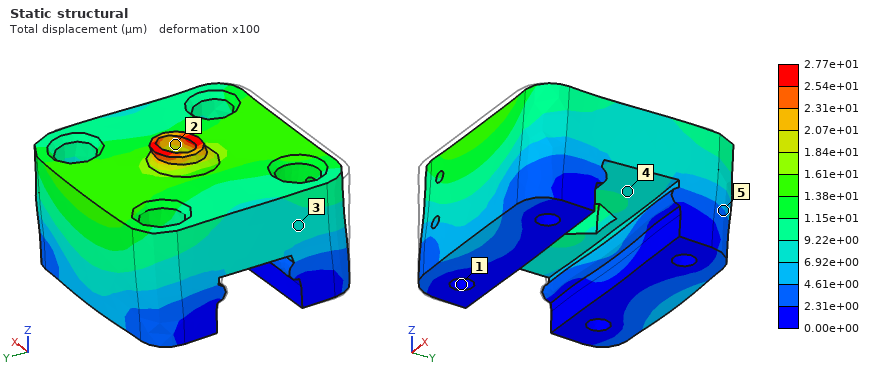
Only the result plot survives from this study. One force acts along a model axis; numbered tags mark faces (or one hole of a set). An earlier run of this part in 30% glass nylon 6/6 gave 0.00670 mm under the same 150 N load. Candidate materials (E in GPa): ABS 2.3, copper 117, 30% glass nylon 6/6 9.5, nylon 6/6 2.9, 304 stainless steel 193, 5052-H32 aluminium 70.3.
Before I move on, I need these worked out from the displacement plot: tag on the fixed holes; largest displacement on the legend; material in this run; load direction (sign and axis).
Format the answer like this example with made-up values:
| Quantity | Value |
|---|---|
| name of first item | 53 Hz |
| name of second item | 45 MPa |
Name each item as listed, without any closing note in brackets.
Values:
| Quantity | Value |
|---|---|
| tag on the fixed holes | 1 |
| largest displacement on the legend | 2.77e+01 µm |
| material in this run | ABS |
| load direction | +Y |
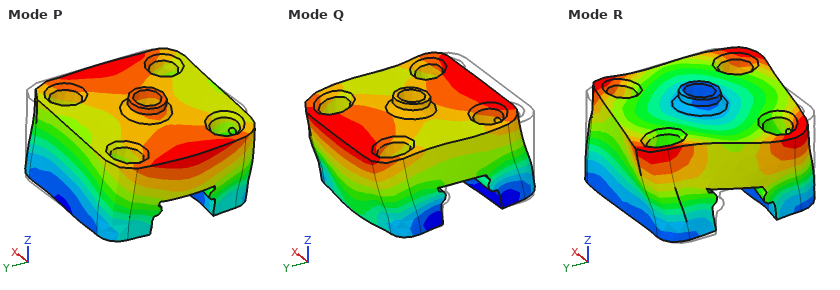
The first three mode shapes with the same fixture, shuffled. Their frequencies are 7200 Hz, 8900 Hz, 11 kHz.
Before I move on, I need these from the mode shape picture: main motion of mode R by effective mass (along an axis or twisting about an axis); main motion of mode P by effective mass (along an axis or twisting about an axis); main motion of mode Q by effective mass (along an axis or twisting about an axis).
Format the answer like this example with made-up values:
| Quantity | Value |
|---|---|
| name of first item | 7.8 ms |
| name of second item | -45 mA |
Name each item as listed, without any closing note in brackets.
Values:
| Quantity | Value |
|---|---|
| main motion of mode R by effective mass | twisting about Z |
| main motion of mode P by effective mass | along X |
| main motion of mode Q by effective mass | along Y |
